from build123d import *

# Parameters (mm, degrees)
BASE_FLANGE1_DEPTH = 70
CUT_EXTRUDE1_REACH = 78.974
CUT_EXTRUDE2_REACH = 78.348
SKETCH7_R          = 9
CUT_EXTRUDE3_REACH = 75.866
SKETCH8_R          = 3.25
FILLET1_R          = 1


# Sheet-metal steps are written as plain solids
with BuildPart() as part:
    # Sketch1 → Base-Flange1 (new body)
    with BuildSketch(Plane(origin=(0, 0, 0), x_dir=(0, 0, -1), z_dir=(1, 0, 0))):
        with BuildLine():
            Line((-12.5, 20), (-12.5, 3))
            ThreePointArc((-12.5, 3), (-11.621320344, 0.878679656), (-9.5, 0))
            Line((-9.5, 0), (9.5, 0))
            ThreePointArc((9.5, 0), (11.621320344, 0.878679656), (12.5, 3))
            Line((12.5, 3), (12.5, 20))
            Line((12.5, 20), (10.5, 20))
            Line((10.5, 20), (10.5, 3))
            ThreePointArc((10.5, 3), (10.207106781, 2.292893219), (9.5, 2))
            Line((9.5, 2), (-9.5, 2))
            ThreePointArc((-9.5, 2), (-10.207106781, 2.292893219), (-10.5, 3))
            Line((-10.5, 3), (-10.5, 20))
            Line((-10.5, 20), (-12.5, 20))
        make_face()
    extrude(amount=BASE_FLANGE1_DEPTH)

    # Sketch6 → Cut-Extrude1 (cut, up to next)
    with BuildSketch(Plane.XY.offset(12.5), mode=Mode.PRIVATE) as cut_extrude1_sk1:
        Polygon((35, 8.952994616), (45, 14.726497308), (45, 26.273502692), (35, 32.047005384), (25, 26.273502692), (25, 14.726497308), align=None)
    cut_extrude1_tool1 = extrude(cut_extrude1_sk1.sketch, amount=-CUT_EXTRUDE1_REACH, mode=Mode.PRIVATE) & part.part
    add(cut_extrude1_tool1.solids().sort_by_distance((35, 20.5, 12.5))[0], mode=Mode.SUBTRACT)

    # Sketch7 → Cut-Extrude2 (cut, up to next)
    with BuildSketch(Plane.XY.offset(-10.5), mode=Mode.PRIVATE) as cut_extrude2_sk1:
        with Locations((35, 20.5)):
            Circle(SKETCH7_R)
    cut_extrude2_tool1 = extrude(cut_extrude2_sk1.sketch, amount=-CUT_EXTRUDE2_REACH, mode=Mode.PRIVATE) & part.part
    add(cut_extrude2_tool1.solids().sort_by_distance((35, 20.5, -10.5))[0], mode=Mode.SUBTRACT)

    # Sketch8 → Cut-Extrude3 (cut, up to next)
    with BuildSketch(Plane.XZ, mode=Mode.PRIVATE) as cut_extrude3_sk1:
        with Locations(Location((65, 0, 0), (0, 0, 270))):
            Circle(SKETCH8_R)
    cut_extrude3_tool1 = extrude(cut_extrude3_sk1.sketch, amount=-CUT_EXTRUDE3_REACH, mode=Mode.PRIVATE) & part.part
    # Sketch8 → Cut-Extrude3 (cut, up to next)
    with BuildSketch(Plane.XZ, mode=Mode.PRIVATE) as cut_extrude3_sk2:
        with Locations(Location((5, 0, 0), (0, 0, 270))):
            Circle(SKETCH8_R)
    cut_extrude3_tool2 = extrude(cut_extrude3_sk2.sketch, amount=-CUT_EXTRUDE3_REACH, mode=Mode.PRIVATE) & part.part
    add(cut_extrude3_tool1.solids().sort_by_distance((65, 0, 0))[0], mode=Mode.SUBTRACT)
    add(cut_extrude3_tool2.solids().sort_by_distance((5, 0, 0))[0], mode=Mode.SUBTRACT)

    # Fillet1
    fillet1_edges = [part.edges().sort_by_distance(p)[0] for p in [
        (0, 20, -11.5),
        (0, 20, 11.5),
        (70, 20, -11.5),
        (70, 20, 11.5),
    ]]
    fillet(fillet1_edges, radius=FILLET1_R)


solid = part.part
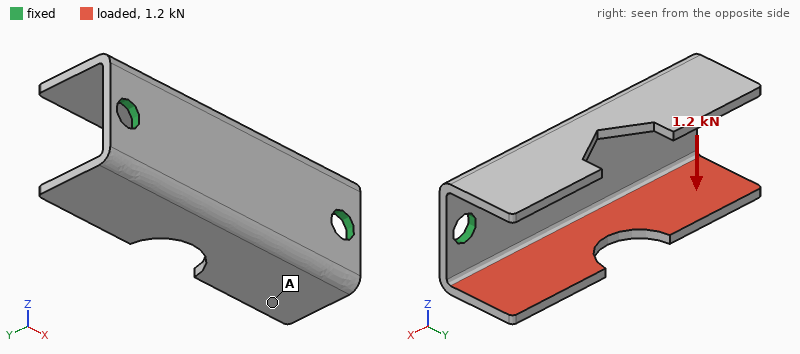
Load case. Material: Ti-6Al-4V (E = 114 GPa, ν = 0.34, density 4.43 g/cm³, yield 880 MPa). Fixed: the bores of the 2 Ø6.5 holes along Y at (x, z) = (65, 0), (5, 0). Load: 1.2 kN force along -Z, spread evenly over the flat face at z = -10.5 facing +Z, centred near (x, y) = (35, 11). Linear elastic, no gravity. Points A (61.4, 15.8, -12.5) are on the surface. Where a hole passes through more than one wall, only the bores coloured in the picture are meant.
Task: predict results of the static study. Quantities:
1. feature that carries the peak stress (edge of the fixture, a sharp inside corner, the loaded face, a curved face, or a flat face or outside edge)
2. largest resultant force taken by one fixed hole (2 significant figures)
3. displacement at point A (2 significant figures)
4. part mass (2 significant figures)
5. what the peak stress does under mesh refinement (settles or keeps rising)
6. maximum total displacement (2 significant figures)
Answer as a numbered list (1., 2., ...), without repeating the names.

1. edge of the fixture
2. 600 N
3. 0.51 mm
4. 34 g
5. keeps rising
6. 0.66 mm
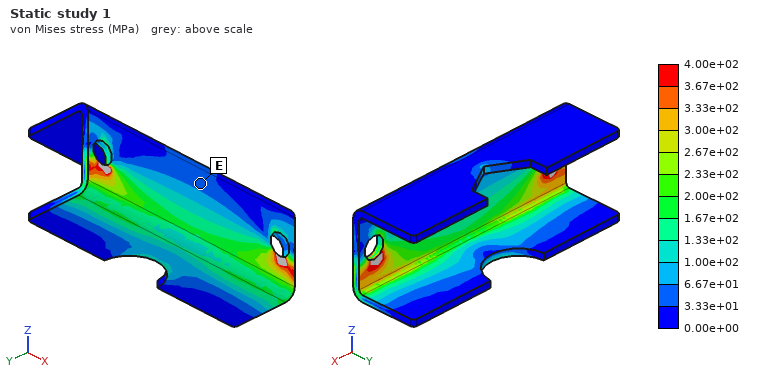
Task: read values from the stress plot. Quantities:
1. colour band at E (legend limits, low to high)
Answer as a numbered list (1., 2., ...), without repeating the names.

1. 3.33e+01 to 6.67e+01 MPa
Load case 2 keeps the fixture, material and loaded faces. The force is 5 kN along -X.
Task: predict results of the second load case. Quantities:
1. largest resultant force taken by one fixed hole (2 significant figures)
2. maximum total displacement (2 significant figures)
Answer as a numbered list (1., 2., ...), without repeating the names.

1. 2.8 kN
2. 0.46 mm
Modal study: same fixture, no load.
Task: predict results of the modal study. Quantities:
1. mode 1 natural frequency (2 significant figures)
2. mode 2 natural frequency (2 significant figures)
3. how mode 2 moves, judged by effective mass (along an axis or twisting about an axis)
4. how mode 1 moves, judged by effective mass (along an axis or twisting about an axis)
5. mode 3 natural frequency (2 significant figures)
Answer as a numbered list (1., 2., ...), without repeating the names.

1. 2400 Hz
2. 2800 Hz
3. along Y
4. along Z
5. 3300 Hz
